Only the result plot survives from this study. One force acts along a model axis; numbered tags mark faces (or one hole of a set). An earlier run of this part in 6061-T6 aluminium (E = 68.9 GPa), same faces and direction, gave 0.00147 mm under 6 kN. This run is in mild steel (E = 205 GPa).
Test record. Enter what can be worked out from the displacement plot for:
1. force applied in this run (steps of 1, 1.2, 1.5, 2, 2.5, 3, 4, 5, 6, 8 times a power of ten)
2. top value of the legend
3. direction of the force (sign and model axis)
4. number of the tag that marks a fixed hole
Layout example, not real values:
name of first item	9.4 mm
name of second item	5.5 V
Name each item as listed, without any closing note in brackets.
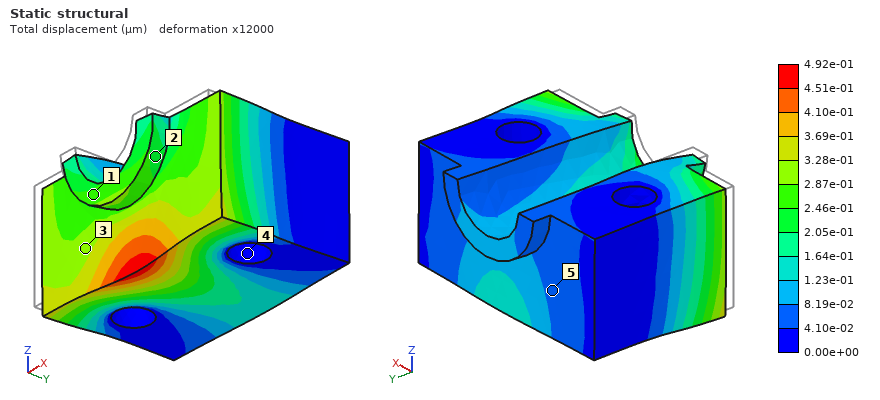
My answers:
force applied in this run	6 kN
top value of the legend	4.92e-01 µm
direction of the force	+Y
number of the tag that marks a fixed hole	4
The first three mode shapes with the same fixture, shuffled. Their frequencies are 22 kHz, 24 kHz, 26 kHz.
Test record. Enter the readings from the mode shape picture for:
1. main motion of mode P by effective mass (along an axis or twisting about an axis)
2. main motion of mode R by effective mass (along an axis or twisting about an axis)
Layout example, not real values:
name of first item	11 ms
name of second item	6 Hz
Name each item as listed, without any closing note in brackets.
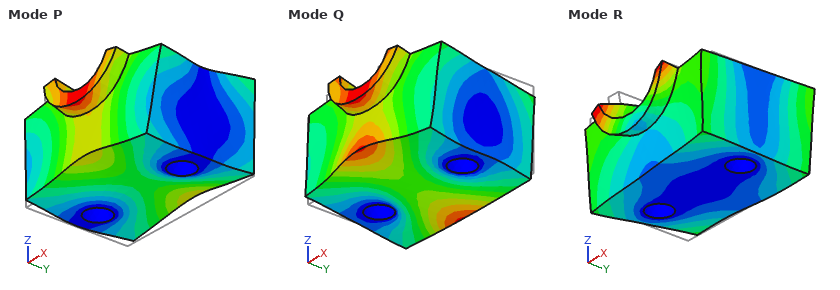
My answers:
main motion of mode P by effective mass	along Z
main motion of mode R by effective mass	twisting about Z
